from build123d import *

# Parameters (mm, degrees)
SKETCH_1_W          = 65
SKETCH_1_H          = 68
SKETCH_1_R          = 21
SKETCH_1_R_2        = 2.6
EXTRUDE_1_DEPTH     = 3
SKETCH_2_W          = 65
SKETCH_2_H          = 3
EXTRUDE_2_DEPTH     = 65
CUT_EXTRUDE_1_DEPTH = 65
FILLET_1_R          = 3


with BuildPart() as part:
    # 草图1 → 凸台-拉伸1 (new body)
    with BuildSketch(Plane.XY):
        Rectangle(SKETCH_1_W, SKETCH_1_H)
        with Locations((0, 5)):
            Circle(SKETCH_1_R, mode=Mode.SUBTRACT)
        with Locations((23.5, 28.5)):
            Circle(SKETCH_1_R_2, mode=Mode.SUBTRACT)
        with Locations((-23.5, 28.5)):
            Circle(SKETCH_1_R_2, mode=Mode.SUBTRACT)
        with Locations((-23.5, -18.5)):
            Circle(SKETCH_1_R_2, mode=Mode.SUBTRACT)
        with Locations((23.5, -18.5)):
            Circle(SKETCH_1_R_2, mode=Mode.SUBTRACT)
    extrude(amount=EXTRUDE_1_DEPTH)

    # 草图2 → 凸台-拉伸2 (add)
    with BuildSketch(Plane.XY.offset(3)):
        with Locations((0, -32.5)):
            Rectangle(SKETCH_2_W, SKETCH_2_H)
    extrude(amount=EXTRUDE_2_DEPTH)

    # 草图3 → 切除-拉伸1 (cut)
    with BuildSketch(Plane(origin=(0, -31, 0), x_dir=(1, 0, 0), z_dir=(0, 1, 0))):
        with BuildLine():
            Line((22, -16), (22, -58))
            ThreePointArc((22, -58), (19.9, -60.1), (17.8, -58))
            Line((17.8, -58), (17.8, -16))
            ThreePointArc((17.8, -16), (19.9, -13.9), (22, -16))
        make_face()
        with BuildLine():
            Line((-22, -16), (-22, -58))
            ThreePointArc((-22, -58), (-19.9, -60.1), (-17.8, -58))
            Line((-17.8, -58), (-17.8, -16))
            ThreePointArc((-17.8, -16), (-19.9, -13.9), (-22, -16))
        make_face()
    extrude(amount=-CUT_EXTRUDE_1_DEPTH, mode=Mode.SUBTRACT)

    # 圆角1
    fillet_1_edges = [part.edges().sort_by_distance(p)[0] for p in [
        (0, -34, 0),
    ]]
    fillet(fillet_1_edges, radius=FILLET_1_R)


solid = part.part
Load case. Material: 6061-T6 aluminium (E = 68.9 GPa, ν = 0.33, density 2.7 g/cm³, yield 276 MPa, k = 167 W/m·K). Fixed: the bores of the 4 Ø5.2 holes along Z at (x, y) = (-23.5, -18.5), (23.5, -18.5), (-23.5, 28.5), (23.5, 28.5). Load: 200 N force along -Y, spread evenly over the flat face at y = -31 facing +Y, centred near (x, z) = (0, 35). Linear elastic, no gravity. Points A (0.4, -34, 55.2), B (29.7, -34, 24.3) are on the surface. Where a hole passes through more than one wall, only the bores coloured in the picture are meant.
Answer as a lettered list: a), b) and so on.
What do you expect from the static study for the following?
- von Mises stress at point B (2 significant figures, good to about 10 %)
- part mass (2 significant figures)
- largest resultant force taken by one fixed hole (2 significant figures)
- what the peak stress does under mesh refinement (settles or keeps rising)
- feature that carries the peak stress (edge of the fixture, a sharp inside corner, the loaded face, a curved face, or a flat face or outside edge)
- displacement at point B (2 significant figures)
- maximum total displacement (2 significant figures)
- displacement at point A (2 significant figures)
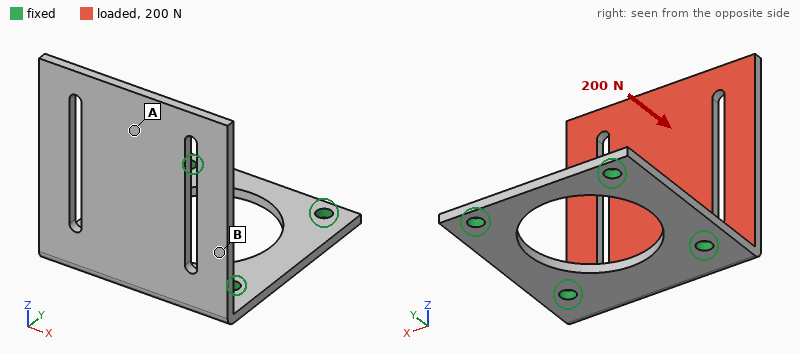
a) 37 MPa
b) 55 g
c) 110 N
d) keeps rising
e) edge of the fixture
f) 0.35 mm
g) 1.4 mm
h) 1.1 mm
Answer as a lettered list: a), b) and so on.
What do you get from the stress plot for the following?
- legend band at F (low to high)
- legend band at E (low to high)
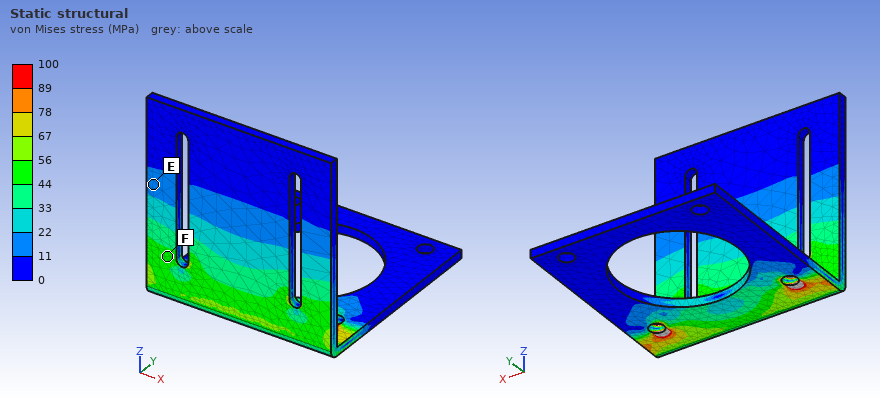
a) 44 to 56 MPa
b) 11 to 22 MPa
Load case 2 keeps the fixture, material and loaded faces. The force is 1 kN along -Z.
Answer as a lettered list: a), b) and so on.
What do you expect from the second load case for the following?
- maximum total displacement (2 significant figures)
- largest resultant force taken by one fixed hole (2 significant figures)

a) 0.34 mm
b) 510 N
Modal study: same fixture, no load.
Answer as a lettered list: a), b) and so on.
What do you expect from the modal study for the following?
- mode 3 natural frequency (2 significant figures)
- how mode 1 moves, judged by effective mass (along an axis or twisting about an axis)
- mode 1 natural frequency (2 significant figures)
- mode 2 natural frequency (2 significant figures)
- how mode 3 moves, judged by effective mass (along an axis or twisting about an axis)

a) 1900 Hz
b) along Y
c) 420 Hz
d) 1200 Hz
e) along X
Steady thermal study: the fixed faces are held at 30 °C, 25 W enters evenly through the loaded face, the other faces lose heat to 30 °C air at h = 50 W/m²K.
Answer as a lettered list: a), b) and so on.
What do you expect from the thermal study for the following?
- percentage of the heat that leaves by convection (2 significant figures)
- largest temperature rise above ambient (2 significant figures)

a) 28 %
b) 31 K
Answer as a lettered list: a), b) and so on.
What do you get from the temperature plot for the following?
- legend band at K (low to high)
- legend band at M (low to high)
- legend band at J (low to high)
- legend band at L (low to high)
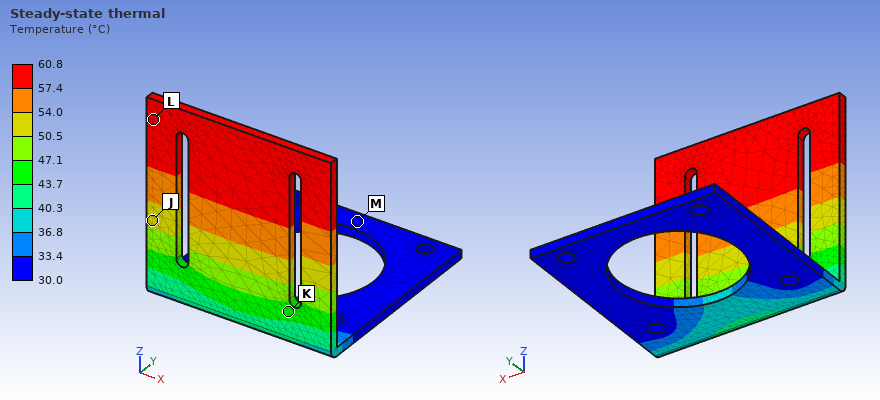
a) 43.7 to 47.1 °C
b) 30.0 to 33.4 °C
c) 50.5 to 54.0 °C
d) 57.4 to 60.8 °C
